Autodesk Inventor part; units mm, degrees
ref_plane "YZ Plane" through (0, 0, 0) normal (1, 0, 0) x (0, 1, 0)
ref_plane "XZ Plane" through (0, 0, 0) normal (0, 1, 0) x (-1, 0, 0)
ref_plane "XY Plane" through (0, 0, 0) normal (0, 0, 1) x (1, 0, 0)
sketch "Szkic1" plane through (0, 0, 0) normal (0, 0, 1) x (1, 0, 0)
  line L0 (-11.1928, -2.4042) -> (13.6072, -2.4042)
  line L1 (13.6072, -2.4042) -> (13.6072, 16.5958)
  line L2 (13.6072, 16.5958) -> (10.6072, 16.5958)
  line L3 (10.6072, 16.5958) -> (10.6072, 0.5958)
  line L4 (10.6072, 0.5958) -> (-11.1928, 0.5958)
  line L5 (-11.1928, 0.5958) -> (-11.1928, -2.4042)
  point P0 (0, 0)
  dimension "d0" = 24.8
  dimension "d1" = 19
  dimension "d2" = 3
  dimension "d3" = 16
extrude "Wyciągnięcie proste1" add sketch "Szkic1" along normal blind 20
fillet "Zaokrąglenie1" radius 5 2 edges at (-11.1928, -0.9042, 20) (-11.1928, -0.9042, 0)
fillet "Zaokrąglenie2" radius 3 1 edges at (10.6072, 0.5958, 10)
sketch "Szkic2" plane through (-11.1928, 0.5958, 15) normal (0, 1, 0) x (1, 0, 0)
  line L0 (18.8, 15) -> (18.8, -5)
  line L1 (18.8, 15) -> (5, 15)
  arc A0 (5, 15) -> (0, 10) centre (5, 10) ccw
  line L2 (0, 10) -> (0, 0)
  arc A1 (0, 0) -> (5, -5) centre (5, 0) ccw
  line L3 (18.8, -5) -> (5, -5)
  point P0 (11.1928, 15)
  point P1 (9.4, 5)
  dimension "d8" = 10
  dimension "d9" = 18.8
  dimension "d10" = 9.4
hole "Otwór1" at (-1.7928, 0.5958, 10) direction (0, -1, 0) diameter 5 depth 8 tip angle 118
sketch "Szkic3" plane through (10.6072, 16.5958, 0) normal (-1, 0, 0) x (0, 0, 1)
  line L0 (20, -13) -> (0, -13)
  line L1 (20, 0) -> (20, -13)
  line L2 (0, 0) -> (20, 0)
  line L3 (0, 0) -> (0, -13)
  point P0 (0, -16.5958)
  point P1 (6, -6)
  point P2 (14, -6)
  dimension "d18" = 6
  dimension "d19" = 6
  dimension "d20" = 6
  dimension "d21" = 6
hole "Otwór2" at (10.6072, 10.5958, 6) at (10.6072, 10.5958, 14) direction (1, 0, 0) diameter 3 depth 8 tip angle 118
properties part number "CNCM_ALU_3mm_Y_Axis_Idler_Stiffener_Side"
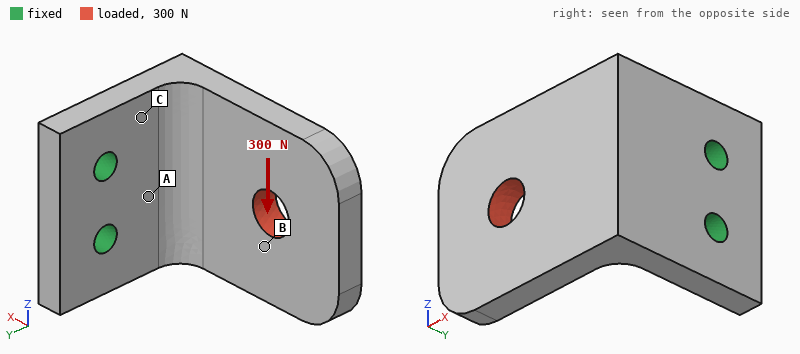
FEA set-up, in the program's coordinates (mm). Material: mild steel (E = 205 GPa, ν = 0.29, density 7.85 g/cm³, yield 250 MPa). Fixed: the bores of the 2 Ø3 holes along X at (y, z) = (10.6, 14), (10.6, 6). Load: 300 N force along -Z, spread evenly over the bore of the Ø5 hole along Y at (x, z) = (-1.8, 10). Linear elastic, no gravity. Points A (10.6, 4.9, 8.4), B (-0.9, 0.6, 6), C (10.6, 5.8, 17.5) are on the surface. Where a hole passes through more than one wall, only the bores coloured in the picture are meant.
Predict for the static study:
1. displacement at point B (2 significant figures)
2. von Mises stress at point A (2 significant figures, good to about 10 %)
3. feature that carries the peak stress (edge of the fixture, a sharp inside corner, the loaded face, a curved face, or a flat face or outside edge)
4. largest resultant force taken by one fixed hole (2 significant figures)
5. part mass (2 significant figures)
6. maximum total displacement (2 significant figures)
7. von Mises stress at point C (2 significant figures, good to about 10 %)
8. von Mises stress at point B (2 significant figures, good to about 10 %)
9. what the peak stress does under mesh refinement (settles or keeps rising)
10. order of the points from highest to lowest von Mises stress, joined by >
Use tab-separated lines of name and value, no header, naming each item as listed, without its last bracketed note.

displacement at point B	23 µm
von Mises stress at point A	81 MPa
feature that carries the peak stress	edge of the fixture
largest resultant force taken by one fixed hole	480 N
part mass	18 g
maximum total displacement	39 µm
von Mises stress at point C	53 MPa
von Mises stress at point B	16 MPa
what the peak stress does under mesh refinement	keeps rising
order of the points from highest to lowest von Mises stress, joined by >	A > C > B
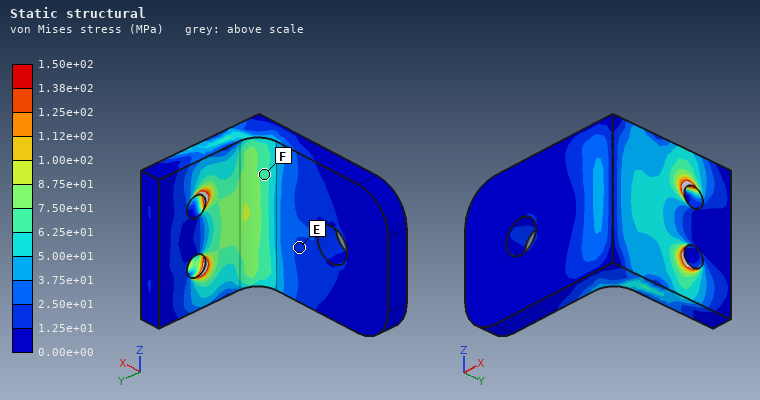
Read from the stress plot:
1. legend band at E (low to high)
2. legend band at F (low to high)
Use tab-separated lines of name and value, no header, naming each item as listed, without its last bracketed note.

legend band at E	1.25e+01 to 2.50e+01 MPa
legend band at F	6.25e+01 to 7.50e+01 MPa
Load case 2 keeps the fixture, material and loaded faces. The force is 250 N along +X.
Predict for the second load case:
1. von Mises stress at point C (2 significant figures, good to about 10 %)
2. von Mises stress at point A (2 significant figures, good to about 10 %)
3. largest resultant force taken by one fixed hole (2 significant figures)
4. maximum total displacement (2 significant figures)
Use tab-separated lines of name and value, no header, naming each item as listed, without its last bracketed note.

von Mises stress at point C	49 MPa
von Mises stress at point A	45 MPa
largest resultant force taken by one fixed hole	130 N
maximum total displacement	39 µm
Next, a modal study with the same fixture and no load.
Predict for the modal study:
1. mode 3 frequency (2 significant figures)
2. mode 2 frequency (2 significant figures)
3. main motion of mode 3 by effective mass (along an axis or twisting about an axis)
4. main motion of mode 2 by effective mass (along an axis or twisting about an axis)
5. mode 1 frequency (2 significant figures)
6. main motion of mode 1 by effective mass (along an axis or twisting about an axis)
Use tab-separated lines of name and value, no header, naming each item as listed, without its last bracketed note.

mode 3 frequency	10 kHz
mode 2 frequency	5500 Hz
main motion of mode 3 by effective mass	along X
main motion of mode 2 by effective mass	along Z
mode 1 frequency	3000 Hz
main motion of mode 1 by effective mass	along Y
